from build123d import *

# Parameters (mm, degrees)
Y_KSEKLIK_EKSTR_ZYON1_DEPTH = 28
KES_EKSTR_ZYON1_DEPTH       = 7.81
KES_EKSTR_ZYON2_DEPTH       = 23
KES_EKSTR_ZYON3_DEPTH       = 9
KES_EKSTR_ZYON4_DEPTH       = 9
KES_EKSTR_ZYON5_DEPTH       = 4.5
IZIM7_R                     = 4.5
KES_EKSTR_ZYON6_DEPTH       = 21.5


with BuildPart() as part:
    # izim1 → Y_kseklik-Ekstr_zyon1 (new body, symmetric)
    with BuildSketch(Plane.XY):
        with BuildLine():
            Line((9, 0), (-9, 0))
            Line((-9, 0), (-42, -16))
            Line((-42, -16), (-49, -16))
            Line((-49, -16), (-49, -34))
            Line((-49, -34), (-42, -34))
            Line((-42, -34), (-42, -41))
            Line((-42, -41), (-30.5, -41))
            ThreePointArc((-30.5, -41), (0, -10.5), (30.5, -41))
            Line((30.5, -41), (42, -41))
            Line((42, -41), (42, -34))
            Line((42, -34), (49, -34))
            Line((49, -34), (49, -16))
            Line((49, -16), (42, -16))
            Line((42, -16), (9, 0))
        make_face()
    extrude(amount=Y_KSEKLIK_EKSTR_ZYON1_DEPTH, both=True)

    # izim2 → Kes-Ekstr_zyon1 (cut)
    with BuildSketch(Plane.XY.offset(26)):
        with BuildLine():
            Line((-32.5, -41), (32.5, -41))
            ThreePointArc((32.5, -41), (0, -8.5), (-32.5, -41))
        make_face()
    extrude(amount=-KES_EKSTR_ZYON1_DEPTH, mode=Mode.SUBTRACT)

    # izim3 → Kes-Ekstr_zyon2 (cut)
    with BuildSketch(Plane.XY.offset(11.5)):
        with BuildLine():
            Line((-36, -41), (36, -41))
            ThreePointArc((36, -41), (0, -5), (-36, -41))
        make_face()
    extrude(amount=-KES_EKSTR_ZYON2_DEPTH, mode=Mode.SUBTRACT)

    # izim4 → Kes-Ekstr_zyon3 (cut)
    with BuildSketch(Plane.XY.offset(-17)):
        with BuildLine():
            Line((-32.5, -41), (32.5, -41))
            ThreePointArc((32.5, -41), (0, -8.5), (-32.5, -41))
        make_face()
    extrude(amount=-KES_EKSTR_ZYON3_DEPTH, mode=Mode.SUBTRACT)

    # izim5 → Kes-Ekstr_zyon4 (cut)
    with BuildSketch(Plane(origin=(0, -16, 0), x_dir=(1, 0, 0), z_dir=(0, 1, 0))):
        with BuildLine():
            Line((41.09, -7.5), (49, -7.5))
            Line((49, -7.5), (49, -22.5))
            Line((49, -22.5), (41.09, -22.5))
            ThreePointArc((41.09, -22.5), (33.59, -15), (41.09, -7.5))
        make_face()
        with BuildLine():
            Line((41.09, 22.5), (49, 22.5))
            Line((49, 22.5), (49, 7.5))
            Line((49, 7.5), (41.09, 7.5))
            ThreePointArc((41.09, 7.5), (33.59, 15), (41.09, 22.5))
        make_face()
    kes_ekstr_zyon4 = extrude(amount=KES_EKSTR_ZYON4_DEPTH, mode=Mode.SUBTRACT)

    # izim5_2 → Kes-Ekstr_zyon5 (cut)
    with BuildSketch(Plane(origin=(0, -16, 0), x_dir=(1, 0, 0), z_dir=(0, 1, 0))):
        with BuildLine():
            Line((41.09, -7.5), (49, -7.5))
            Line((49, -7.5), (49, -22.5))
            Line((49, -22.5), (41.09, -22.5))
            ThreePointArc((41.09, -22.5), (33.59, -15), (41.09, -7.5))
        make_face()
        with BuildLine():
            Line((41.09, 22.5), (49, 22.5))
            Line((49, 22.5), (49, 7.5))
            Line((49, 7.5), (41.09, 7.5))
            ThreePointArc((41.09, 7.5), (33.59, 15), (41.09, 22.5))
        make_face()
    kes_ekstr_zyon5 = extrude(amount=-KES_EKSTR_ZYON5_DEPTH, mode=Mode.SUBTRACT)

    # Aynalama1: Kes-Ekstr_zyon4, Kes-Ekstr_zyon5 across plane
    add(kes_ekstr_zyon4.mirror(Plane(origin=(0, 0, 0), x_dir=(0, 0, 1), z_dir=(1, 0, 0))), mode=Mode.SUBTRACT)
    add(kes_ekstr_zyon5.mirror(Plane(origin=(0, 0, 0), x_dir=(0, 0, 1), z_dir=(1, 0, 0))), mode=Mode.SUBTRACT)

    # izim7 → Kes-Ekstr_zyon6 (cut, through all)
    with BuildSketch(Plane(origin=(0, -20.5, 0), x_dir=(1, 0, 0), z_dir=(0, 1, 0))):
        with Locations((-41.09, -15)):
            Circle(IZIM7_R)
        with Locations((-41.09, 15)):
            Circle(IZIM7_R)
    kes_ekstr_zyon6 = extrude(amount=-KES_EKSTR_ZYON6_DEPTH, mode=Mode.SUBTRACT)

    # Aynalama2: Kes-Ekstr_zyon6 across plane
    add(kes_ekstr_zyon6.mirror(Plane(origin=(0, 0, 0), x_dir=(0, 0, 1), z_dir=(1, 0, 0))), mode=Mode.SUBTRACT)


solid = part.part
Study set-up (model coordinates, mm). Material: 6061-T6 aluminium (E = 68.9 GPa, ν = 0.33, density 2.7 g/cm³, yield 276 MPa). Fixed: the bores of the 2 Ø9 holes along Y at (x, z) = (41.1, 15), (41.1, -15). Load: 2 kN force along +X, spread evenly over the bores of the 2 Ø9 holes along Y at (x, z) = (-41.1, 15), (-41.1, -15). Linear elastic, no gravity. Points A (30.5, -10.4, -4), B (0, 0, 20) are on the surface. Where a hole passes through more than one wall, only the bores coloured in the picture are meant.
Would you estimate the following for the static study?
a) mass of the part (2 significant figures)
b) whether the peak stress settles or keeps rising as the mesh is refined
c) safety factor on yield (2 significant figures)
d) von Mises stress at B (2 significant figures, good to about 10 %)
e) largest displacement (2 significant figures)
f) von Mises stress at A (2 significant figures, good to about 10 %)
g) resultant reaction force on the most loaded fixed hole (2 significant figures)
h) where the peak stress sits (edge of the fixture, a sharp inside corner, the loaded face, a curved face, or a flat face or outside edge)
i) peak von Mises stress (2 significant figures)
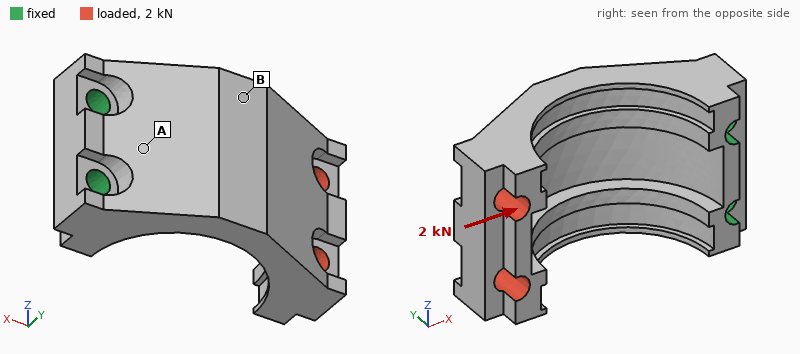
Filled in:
190 g
settles
2.3
63 MPa
0.65 mm
21 MPa
1.0 kN
a curved face
120 MPa
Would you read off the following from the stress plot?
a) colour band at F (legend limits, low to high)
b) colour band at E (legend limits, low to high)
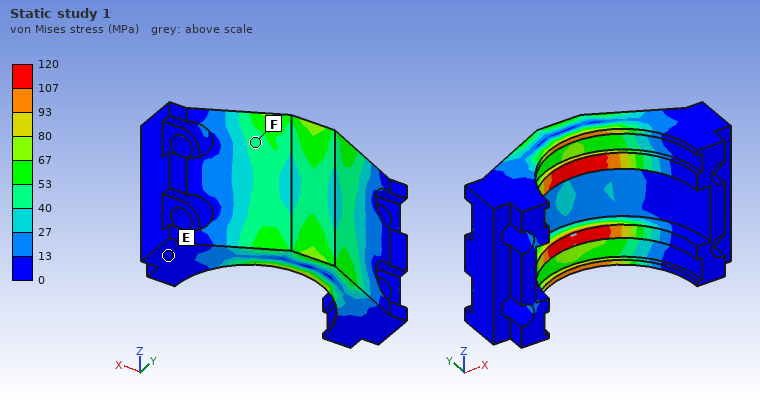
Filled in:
40 to 53 MPa
0 to 13 MPa
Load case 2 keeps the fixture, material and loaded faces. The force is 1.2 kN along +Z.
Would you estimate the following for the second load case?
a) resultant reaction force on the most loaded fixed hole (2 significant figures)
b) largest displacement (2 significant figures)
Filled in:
2.1 kN
0.40 mm
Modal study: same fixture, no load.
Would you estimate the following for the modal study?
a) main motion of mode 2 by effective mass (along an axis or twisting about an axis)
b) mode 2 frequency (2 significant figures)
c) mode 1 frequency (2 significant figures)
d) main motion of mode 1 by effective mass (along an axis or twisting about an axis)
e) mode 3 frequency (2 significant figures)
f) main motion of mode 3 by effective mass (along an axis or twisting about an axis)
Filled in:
along Z
1300 Hz
770 Hz
along Y
2900 Hz
along X
